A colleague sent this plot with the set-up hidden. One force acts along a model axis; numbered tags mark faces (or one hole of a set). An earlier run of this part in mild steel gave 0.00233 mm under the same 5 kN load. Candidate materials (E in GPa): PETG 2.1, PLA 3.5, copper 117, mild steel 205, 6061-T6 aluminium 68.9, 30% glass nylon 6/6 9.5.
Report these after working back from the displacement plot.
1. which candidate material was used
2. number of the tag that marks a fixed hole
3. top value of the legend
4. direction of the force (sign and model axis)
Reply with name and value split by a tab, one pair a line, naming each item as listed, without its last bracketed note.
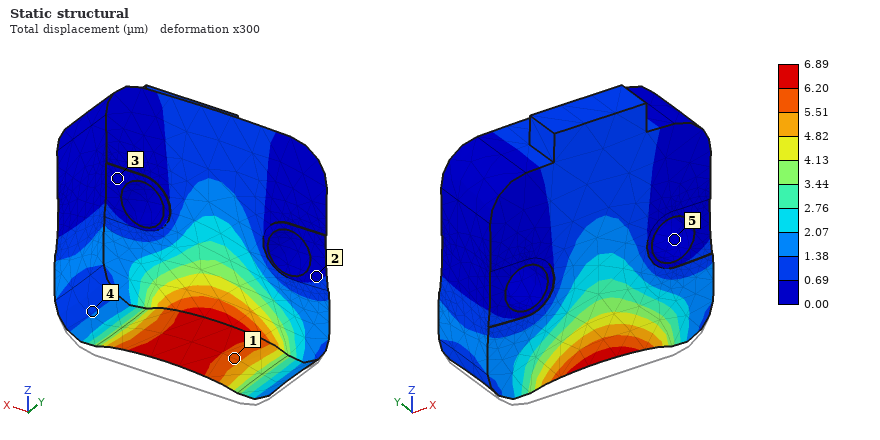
which candidate material was used	6061-T6 aluminium
number of the tag that marks a fixed hole	5
top value of the legend	6.89 µm
direction of the force	+Z
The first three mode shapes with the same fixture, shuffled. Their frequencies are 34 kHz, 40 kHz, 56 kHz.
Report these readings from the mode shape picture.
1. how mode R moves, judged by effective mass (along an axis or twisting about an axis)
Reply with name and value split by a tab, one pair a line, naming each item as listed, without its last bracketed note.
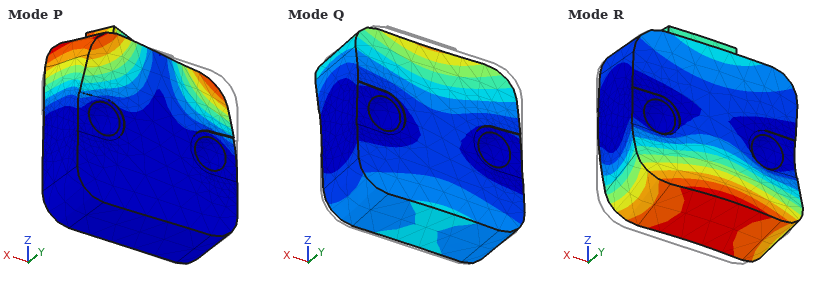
how mode R moves, judged by effective mass	along Y
